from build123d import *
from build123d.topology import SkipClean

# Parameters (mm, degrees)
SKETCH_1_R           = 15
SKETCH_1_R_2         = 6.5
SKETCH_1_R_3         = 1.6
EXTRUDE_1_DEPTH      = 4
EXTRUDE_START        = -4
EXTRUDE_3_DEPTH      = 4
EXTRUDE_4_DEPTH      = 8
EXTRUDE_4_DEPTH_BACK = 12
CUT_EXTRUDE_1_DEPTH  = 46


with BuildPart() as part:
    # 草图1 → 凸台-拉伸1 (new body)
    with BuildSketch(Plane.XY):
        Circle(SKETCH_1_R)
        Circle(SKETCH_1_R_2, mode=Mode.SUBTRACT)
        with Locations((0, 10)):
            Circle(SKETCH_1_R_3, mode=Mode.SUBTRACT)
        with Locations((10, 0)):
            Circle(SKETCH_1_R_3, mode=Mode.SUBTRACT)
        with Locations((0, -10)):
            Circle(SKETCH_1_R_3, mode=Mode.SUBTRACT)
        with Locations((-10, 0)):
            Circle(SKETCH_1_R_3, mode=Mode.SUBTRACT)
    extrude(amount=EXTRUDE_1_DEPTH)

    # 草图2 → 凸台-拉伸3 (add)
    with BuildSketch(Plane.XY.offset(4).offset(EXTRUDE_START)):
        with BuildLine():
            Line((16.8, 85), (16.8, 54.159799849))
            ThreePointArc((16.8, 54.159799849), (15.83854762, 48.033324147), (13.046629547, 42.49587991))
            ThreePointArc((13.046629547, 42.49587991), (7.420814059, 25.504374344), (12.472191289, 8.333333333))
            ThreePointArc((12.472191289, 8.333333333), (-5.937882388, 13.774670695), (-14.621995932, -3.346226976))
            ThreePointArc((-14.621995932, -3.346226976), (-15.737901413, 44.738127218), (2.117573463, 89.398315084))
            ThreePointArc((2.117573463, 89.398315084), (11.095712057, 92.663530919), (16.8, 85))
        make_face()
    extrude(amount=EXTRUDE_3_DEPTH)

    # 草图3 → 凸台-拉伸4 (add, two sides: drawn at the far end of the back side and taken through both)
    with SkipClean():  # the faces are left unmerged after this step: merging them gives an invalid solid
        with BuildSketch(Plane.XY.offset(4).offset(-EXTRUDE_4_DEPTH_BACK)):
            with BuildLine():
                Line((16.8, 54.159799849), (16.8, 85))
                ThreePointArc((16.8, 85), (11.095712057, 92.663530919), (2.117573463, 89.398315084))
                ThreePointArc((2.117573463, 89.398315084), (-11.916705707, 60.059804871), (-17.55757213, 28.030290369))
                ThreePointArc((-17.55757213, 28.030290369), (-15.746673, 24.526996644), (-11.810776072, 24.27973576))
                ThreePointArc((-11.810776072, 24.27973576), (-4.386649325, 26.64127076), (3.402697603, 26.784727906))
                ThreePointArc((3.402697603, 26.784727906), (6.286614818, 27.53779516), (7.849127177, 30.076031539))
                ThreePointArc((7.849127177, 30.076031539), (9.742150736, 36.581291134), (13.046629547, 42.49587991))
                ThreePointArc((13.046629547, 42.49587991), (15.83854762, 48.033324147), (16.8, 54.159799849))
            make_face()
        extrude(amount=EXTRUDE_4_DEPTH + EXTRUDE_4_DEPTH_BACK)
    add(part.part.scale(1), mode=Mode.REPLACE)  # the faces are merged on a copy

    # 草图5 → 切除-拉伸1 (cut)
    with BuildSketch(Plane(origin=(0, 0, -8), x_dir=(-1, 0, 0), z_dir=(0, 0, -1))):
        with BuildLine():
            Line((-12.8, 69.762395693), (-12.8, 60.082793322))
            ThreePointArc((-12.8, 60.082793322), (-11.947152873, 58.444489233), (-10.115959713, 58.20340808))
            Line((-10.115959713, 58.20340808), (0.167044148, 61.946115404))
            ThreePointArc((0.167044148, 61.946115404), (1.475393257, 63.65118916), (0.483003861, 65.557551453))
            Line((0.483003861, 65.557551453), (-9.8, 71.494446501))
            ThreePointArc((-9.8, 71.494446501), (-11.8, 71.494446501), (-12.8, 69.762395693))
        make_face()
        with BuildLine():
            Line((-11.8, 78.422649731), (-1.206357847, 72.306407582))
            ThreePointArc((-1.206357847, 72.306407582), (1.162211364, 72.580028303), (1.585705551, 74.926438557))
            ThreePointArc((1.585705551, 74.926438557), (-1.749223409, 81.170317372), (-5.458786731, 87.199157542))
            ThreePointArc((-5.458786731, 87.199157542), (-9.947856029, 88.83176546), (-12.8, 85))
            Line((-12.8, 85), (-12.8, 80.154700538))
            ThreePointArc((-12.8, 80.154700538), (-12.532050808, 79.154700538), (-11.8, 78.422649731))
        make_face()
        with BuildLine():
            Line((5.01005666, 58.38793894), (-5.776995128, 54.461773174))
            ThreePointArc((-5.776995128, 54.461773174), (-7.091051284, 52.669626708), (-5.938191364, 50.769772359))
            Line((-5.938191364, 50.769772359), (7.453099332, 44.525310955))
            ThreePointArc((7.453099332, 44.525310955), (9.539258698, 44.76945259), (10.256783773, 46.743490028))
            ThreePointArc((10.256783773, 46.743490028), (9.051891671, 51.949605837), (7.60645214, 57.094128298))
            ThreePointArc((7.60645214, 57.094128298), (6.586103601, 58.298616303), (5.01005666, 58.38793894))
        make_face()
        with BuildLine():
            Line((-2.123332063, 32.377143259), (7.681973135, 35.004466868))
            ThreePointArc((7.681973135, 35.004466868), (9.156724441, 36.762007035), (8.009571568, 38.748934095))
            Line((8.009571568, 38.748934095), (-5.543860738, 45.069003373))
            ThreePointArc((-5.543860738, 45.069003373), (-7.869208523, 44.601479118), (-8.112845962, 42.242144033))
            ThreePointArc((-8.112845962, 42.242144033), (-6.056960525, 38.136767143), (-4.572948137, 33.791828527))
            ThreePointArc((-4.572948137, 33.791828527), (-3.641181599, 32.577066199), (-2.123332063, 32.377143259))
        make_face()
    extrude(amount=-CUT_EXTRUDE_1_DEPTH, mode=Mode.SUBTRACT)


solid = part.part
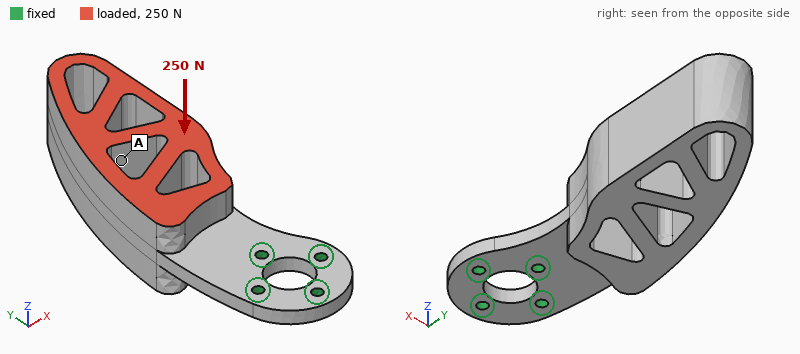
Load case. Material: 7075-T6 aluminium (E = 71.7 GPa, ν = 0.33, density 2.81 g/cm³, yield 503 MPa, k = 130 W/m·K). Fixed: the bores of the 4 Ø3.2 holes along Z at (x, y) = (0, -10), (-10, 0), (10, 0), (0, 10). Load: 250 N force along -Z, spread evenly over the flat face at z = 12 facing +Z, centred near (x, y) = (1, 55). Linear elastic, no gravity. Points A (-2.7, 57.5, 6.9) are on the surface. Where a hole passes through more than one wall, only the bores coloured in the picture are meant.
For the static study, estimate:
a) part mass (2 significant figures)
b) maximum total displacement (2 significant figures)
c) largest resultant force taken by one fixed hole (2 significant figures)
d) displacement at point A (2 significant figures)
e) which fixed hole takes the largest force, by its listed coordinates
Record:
73 g
1.2 mm
740 N
0.65 mm
(0, 10)
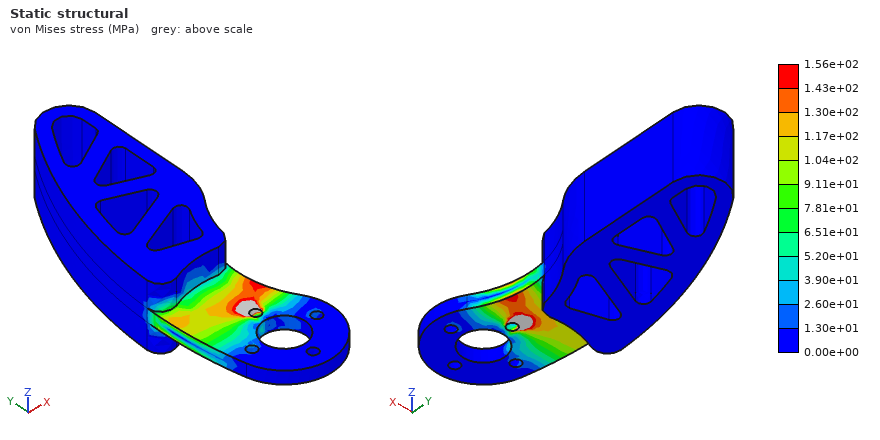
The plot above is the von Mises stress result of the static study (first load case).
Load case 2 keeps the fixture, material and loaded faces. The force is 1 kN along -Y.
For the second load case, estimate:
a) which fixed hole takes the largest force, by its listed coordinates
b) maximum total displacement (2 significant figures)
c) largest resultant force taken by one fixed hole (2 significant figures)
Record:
(0, 10)
1.3 mm
810 N
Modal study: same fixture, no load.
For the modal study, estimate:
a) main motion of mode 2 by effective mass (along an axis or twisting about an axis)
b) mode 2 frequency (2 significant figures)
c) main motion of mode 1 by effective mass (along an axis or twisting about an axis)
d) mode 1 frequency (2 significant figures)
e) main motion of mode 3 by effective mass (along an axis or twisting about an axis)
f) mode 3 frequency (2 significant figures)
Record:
along X
1600 Hz
along Z
370 Hz
twisting about Y
1900 Hz
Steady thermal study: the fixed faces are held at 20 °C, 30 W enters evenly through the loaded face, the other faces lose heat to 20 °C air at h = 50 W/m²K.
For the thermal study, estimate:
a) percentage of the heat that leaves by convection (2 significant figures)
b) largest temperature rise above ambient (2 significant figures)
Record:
47 %
38 K
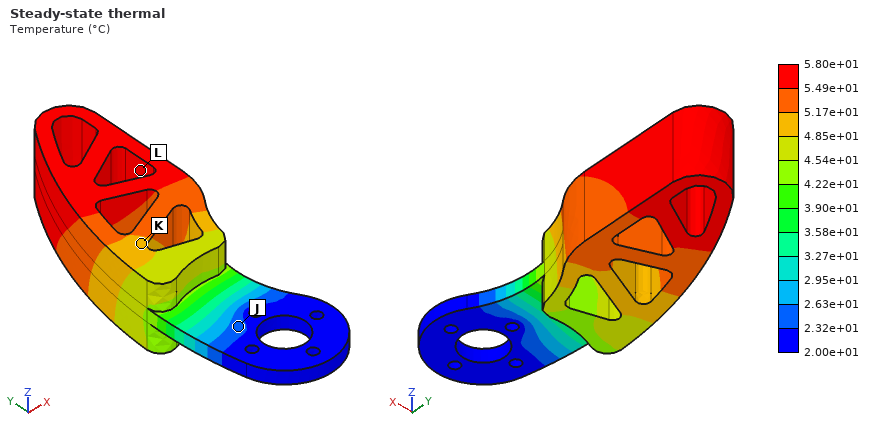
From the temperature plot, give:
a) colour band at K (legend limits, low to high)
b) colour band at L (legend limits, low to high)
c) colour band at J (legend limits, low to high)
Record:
4.85e+01 to 5.17e+01 °C
5.49e+01 to 5.80e+01 °C
2.32e+01 to 2.63e+01 °C
